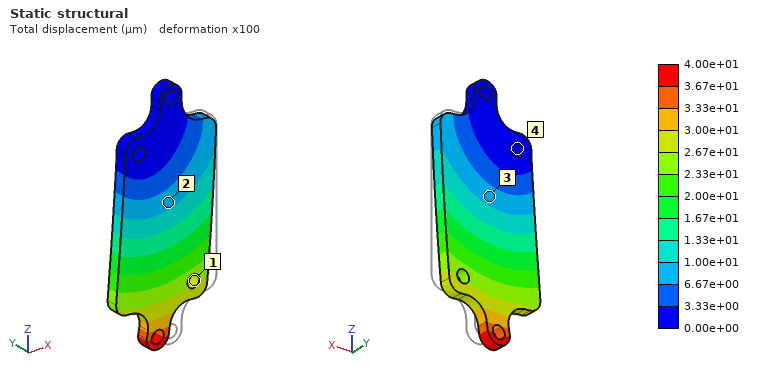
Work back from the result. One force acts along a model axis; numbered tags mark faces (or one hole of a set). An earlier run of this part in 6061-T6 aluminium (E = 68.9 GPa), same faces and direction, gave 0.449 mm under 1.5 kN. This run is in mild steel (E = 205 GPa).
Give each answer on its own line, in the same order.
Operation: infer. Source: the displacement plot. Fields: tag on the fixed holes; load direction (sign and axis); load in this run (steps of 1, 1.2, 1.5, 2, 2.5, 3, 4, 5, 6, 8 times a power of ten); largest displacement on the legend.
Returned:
4
-X
400 N
4.00e+01 µm
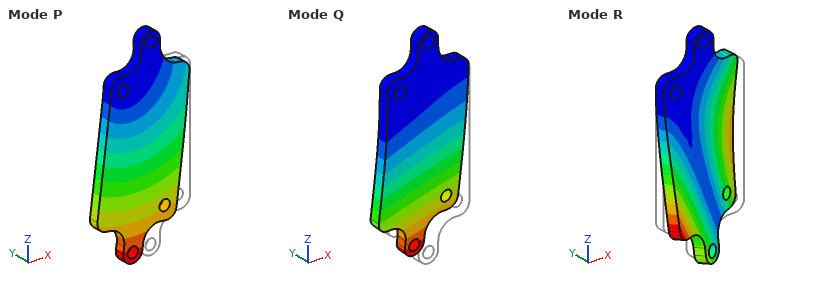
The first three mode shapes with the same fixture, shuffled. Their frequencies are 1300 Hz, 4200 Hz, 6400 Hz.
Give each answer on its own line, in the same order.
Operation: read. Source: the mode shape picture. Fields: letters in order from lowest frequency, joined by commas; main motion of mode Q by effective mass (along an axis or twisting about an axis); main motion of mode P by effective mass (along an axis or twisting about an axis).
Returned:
Q, R, P
along Y
along X
